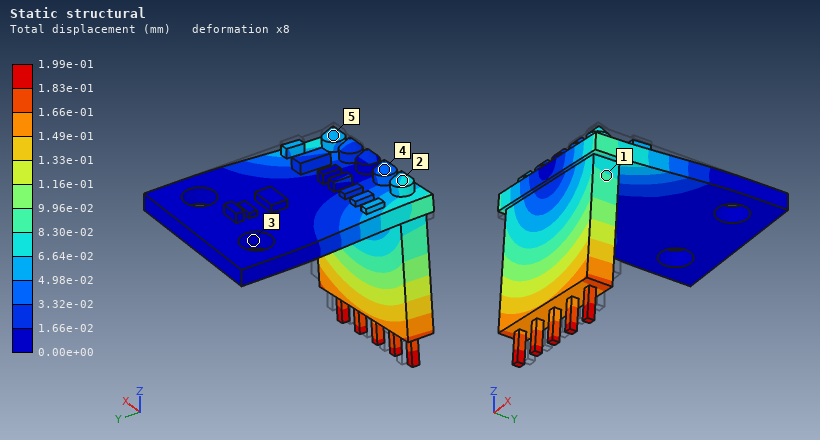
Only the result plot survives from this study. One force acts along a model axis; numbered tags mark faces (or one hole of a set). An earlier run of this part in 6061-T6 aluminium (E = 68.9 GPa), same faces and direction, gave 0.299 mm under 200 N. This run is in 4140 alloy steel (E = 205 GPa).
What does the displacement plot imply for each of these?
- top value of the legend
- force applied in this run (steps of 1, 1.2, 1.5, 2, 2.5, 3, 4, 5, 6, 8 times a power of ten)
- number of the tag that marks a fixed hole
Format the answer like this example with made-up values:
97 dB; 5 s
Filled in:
1.99e-01 mm; 400 N; 3
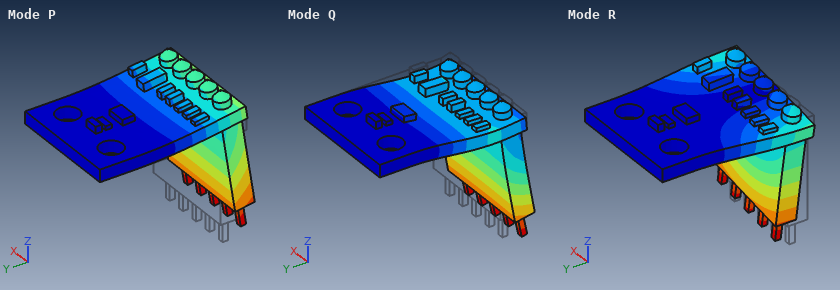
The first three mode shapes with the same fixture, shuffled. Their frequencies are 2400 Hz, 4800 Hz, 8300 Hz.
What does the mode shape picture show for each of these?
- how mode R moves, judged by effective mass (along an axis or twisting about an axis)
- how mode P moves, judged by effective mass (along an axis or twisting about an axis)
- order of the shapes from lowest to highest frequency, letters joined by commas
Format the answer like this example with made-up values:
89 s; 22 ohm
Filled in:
along X; along Z; P, R, Q
